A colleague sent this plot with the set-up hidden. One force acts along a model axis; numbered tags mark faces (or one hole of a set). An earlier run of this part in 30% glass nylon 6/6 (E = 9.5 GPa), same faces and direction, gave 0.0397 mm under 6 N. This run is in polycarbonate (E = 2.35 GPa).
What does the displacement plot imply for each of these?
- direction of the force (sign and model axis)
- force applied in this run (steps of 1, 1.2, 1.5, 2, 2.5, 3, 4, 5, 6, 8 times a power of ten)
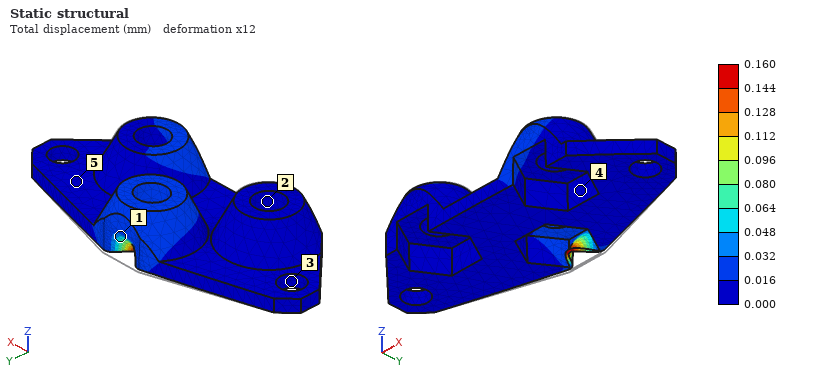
-Y
6 N
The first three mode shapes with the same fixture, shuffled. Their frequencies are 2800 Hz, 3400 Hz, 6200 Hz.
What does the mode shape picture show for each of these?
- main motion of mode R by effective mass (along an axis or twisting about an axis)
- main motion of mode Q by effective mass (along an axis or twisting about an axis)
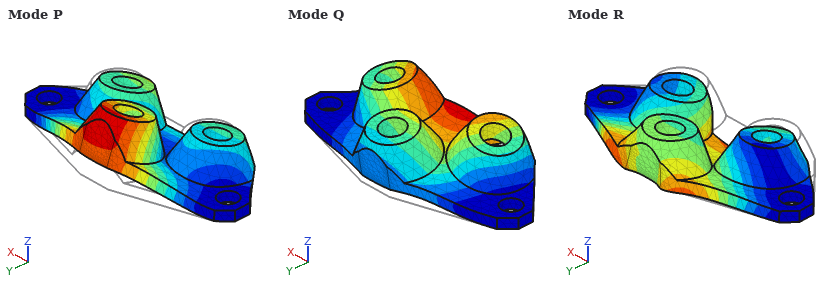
along Y
along Z
